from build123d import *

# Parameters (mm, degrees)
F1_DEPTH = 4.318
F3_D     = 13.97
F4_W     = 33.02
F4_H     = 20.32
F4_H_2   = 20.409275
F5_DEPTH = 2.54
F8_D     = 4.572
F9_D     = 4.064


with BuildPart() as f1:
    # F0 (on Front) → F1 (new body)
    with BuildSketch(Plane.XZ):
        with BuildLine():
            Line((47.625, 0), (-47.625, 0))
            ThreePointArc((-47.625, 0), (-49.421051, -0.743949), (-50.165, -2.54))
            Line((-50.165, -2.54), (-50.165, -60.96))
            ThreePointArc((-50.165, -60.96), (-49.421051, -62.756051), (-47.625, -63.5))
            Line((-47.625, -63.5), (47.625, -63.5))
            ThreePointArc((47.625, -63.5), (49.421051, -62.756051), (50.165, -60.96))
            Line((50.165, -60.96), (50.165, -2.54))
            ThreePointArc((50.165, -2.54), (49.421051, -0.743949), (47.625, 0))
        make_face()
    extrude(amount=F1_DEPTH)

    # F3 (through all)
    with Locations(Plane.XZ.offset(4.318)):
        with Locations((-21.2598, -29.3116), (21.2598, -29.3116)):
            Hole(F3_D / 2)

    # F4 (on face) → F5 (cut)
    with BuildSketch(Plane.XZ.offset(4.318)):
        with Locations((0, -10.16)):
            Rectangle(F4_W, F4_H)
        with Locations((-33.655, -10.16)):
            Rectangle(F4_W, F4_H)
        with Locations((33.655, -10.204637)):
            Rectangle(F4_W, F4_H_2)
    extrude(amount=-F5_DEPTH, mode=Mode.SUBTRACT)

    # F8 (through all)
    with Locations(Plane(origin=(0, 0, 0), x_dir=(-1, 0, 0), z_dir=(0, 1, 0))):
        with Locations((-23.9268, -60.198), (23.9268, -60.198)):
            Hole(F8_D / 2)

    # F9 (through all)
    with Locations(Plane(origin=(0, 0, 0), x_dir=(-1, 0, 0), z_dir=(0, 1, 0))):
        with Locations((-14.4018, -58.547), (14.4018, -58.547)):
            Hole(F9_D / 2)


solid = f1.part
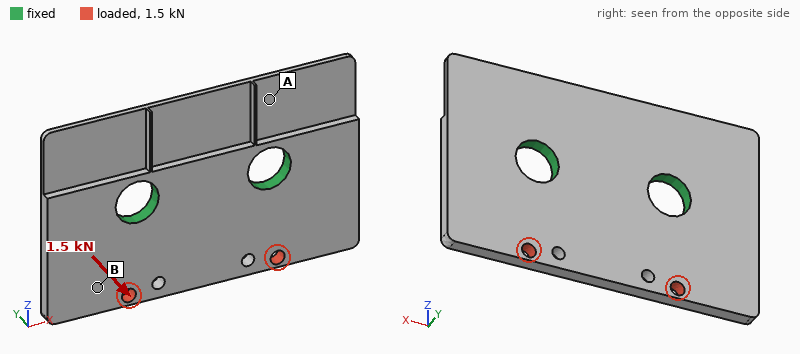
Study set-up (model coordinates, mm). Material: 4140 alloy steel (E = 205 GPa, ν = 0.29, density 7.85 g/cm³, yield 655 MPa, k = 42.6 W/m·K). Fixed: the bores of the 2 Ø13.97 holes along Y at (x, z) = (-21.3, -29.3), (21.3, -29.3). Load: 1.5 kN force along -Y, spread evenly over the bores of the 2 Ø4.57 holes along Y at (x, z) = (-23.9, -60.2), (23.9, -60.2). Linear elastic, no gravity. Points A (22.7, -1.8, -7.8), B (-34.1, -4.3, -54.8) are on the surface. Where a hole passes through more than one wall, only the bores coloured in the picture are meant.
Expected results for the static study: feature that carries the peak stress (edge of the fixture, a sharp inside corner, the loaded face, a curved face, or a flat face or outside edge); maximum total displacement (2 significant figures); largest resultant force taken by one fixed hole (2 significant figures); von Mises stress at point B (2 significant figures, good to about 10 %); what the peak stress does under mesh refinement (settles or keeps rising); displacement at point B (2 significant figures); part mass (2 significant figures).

edge of the fixture
98 µm
750 N
45 MPa
keeps rising
55 µm
160 g
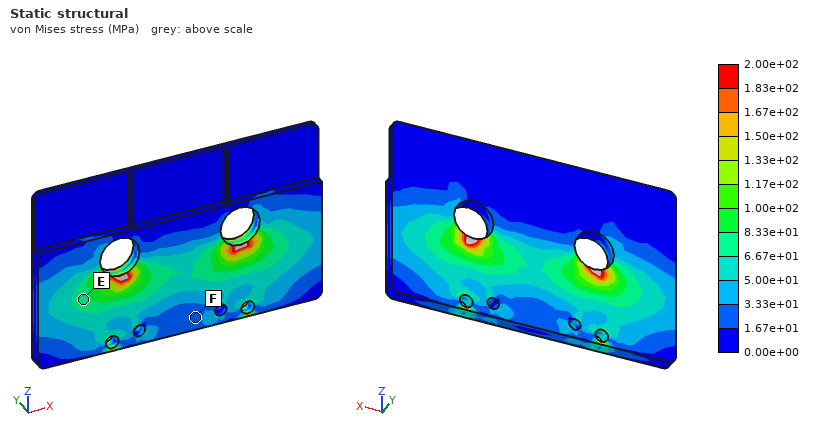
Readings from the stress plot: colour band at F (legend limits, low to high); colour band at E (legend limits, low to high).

1.67e+01 to 3.33e+01 MPa
6.67e+01 to 8.33e+01 MPa
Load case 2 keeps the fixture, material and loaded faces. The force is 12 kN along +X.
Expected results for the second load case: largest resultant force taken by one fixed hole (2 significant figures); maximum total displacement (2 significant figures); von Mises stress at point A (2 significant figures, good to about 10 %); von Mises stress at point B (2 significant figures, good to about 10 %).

8.3 kN
27 µm
21 MPa
42 MPa
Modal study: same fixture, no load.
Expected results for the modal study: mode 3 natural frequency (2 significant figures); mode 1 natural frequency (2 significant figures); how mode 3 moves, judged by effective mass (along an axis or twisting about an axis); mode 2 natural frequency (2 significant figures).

3600 Hz
3400 Hz
along Y
3500 Hz
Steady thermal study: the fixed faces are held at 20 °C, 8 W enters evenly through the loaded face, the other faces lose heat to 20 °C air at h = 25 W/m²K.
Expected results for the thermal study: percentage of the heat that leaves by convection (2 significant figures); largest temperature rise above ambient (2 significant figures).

17 %
22 K
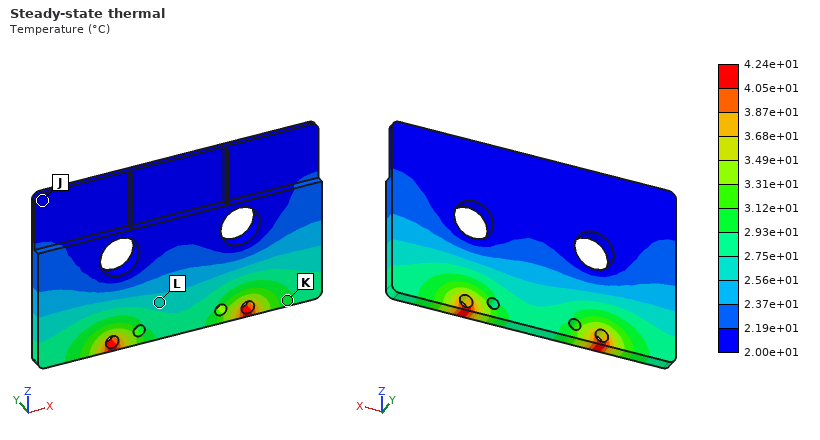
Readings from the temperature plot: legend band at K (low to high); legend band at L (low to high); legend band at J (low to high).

2.93e+01 to 3.12e+01 °C
2.56e+01 to 2.75e+01 °C
2.00e+01 to 2.19e+01 °C
